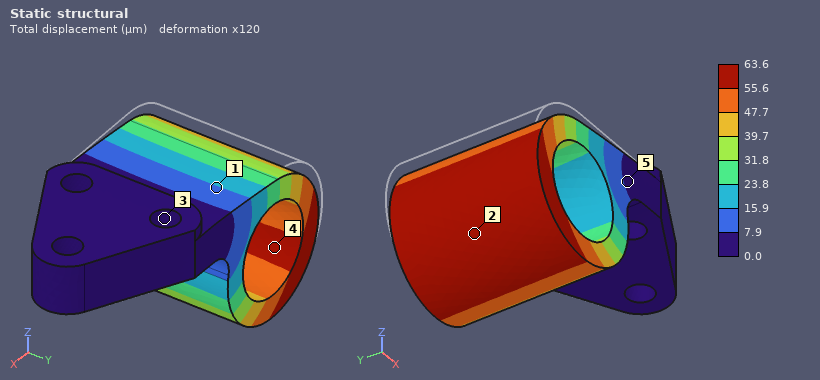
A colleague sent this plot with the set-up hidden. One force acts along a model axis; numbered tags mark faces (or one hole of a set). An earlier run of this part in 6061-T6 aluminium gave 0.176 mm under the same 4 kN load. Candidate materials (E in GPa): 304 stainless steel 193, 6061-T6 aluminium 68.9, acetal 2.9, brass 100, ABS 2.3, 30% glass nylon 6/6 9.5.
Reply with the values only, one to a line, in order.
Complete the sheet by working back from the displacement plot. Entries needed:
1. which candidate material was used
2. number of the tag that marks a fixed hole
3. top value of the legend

304 stainless steel
3
63.6 µm
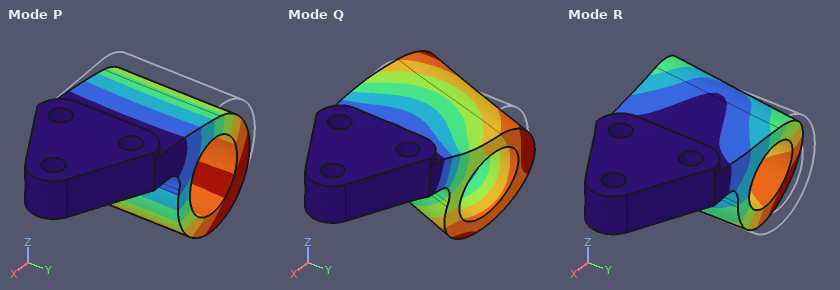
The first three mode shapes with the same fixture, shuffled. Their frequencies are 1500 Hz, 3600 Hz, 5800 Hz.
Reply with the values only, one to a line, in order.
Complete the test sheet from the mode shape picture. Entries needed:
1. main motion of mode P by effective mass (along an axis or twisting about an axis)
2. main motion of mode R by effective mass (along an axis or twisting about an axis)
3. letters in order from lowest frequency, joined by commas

along Z
along Y
P, R, Q
